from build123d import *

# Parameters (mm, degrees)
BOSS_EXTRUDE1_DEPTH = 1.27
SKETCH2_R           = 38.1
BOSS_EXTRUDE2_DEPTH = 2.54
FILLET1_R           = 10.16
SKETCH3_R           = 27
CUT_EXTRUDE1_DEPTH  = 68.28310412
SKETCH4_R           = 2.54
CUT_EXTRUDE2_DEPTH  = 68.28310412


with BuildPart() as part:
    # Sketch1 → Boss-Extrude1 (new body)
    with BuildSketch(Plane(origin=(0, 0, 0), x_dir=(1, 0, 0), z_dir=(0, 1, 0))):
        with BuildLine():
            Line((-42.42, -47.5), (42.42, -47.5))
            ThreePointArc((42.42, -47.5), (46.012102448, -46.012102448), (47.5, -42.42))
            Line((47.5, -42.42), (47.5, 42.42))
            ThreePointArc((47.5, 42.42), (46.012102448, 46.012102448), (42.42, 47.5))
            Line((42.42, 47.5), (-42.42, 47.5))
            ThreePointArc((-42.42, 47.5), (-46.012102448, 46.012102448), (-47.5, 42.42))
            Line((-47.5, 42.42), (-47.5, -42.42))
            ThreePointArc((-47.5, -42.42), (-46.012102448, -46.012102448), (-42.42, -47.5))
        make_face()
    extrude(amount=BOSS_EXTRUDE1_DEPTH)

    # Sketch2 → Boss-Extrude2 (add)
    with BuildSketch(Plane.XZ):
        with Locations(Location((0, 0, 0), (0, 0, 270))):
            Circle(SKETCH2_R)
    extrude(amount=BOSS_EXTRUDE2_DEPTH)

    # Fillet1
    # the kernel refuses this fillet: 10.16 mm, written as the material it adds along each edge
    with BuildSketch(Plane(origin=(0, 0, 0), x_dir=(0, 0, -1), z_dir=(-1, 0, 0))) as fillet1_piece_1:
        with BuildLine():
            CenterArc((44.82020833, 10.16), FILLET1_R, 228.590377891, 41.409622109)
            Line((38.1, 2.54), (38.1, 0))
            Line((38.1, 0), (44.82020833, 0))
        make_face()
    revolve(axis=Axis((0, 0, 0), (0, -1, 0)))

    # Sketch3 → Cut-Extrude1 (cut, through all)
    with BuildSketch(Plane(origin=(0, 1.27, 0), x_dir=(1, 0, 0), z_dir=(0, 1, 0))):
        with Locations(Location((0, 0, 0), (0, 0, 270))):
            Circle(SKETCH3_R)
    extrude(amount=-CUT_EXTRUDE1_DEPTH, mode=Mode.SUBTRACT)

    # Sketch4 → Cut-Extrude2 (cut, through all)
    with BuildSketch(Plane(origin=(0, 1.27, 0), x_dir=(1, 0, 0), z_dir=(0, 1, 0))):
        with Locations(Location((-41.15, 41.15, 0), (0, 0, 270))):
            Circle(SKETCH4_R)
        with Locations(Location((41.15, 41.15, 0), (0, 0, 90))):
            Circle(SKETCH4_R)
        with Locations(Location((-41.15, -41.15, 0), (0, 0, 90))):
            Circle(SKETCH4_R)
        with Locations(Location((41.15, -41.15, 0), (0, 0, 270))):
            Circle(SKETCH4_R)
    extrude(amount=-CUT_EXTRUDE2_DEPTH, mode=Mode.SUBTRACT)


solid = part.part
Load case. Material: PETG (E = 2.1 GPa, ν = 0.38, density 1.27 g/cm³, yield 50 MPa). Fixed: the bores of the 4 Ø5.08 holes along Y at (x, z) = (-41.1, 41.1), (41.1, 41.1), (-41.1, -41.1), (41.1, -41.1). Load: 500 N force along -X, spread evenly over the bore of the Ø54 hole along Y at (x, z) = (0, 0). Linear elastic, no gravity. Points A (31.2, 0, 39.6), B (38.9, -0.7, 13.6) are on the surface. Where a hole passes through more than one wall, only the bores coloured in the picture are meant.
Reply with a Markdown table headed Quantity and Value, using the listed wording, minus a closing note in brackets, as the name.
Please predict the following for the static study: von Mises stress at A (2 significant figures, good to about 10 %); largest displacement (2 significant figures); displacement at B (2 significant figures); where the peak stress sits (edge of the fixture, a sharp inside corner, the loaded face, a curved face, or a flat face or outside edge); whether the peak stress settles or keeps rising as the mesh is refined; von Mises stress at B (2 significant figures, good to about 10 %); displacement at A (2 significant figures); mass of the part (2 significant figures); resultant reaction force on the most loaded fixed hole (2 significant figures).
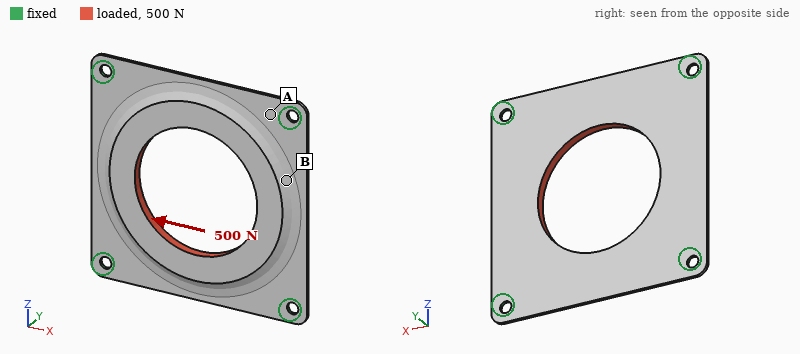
| Quantity | Value |
|---|---|
| von Mises stress at A | 7.0 MPa |
| largest displacement | 0.14 mm |
| displacement at B | 0.11 mm |
| where the peak stress sits | edge of the fixture |
| whether the peak stress settles or keeps rising as the mesh is refined | keeps rising |
| von Mises stress at B | 1.6 MPa |
| displacement at A | 0.063 mm |
| mass of the part | 20 g |
| resultant reaction force on the most loaded fixed hole | 130 N |
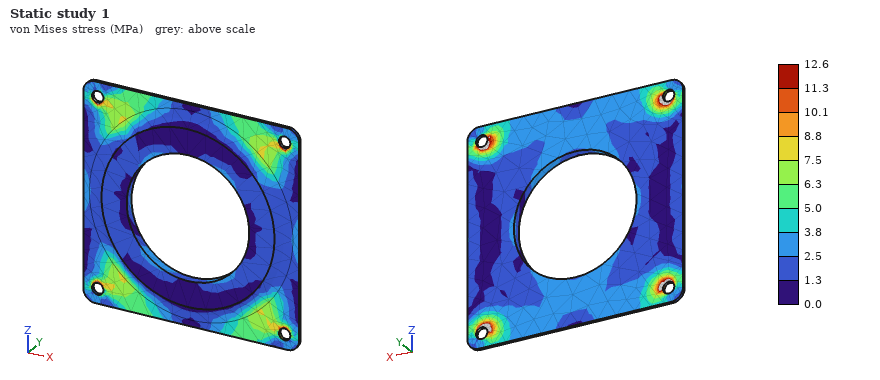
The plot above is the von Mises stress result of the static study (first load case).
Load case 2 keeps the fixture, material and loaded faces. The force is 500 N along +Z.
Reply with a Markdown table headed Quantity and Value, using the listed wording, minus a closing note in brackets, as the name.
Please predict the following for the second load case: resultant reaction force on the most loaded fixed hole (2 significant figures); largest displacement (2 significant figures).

| Quantity | Value |
|---|---|
| resultant reaction force on the most loaded fixed hole | 130 N |
| largest displacement | 0.14 mm |
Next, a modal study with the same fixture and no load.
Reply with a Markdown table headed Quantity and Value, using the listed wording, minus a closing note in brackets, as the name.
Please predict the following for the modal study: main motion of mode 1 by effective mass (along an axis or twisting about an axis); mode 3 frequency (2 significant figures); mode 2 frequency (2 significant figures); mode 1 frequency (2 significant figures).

| Quantity | Value |
|---|---|
| main motion of mode 1 by effective mass | along Y |
| mode 3 frequency | 430 Hz |
| mode 2 frequency | 430 Hz |
| mode 1 frequency | 310 Hz |
